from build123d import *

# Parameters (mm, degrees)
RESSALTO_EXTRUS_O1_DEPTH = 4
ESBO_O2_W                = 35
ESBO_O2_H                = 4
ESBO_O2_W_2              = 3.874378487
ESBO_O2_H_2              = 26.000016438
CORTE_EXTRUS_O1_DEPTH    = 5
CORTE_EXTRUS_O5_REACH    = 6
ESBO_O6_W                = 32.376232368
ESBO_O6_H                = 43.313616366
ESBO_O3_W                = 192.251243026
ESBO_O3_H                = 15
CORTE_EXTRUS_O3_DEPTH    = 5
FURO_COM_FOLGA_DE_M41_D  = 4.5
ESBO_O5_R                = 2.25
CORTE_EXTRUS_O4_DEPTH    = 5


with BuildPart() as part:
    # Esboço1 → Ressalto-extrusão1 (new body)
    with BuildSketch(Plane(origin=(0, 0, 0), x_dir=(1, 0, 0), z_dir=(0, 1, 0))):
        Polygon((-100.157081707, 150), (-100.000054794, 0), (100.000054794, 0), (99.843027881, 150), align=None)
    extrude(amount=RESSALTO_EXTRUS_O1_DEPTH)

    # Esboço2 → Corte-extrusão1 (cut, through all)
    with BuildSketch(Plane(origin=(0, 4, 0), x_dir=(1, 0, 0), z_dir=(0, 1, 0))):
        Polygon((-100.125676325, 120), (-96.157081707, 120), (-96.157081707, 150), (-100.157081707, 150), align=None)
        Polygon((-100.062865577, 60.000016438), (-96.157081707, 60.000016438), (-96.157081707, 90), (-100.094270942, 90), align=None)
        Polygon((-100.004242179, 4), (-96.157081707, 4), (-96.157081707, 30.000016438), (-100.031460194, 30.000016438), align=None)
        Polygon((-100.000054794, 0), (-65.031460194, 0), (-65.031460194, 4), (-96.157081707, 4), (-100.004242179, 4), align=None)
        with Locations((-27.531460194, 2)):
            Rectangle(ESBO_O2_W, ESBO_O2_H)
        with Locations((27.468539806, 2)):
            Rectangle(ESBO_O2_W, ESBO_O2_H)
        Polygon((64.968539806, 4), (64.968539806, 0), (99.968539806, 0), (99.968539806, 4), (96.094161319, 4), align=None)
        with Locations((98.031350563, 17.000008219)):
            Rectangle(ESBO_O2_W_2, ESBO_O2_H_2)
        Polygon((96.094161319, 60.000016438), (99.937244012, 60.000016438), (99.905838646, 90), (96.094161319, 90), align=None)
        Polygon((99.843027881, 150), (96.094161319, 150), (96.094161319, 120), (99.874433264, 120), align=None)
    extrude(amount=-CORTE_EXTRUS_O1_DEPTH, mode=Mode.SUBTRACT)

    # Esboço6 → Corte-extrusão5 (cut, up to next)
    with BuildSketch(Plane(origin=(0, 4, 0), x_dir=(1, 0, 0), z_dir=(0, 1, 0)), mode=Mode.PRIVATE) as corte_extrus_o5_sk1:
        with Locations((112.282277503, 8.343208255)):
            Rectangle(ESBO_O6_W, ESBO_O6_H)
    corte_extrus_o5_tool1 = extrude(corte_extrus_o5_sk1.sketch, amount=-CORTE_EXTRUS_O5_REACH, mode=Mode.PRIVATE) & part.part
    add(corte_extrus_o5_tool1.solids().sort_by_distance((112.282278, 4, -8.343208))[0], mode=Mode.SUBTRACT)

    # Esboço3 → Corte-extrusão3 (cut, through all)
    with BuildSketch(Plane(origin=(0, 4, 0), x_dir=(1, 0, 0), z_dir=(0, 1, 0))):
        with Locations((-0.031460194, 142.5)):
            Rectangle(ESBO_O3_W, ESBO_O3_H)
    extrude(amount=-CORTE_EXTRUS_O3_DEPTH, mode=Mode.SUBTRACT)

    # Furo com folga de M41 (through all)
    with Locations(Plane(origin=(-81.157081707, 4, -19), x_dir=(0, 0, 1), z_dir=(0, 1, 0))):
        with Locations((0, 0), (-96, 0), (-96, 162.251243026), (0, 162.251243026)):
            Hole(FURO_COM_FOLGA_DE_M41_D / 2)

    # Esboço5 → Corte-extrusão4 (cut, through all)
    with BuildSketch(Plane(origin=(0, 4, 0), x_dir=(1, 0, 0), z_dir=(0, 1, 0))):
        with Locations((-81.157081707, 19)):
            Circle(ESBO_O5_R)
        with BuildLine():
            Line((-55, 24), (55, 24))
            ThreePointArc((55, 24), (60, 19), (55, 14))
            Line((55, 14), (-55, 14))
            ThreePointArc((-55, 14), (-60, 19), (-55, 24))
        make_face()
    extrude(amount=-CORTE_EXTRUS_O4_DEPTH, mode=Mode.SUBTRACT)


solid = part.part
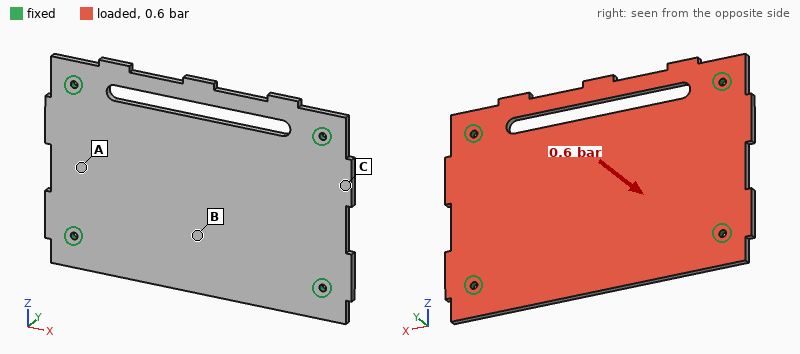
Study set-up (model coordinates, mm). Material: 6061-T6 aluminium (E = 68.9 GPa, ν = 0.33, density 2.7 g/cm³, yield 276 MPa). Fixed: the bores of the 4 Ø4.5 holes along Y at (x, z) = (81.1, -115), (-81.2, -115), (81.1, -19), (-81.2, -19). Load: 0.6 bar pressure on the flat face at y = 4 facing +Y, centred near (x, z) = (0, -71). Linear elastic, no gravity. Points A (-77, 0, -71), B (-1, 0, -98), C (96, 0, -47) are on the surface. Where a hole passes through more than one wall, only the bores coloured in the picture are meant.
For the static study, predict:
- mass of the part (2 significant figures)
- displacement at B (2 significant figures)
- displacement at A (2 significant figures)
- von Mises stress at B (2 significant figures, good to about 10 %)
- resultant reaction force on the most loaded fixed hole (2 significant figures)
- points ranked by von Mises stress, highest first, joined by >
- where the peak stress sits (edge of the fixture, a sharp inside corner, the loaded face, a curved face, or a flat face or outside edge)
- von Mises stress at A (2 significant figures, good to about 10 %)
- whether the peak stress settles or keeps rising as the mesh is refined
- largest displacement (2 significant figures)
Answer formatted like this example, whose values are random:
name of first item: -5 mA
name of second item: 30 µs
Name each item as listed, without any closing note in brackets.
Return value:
mass of the part: 270 g
displacement at B: 0.40 mm
displacement at A: 0.084 mm
von Mises stress at B: 26 MPa
resultant reaction force on the most loaded fixed hole: 400 N
points ranked by von Mises stress, highest first, joined by >: B > A > C
where the peak stress sits: edge of the fixture
von Mises stress at A: 15 MPa
whether the peak stress settles or keeps rising as the mesh is refined: keeps rising
largest displacement: 0.43 mm
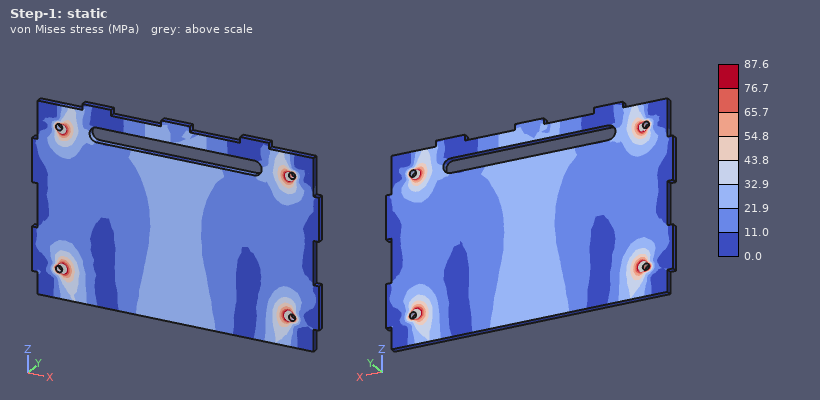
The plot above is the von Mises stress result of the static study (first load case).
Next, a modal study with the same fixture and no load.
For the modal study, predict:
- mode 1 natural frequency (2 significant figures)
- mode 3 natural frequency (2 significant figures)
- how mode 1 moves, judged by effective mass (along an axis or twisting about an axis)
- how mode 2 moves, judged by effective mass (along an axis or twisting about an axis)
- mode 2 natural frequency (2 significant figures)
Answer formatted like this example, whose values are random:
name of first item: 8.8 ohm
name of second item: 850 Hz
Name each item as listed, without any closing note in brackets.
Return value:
mode 1 natural frequency: 670 Hz
mode 3 natural frequency: 1100 Hz
how mode 1 moves, judged by effective mass: along Y
how mode 2 moves, judged by effective mass: twisting about X
mode 2 natural frequency: 940 Hz
